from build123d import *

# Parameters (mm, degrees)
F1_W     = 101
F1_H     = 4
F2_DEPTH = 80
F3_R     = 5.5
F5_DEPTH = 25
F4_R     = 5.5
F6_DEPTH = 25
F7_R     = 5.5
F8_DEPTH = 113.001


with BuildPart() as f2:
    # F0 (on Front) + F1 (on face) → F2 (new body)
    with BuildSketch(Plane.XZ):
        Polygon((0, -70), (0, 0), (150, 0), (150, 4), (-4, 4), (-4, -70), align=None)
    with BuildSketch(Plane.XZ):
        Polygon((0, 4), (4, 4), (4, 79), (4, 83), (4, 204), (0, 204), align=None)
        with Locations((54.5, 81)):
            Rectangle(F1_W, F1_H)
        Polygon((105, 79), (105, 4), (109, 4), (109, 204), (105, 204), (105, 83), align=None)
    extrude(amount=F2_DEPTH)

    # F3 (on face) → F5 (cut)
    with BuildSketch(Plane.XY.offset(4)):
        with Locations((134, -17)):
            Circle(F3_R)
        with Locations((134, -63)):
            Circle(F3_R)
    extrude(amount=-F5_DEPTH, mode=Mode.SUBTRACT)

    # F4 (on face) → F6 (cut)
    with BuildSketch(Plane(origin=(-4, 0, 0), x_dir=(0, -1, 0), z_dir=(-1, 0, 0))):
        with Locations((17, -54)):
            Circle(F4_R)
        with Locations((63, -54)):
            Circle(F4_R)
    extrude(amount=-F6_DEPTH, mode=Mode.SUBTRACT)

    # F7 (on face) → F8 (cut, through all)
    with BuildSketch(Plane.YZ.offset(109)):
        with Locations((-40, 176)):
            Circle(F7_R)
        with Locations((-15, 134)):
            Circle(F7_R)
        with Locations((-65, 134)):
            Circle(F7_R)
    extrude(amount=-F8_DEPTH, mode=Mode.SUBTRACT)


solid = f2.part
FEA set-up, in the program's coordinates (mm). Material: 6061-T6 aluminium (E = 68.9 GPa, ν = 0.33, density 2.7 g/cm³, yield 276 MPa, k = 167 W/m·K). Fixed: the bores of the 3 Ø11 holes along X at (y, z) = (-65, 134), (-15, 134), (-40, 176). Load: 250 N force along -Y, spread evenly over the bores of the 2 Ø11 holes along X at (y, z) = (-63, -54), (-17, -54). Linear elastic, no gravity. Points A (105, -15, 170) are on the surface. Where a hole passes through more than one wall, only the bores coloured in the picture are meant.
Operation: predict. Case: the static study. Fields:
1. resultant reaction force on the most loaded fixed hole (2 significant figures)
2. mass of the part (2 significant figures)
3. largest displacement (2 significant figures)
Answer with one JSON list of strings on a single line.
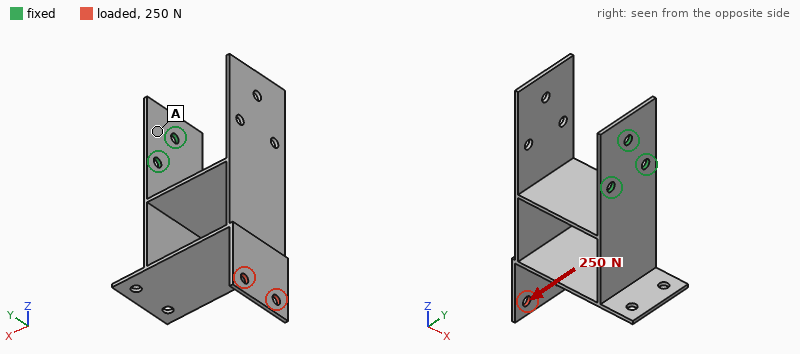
["940 N", "620 g", "3.7 mm"]
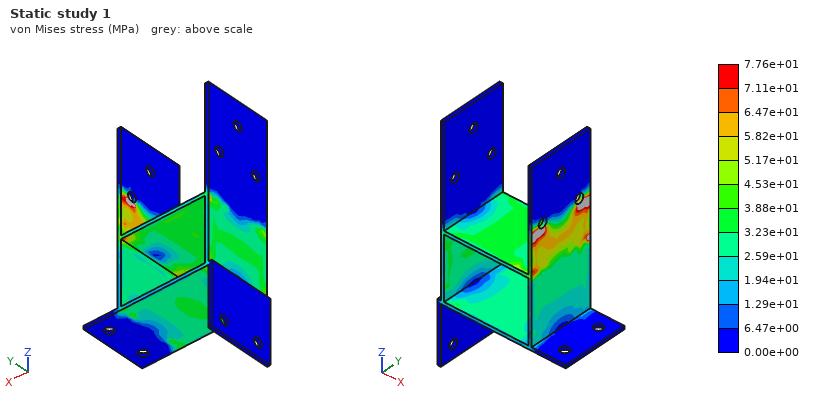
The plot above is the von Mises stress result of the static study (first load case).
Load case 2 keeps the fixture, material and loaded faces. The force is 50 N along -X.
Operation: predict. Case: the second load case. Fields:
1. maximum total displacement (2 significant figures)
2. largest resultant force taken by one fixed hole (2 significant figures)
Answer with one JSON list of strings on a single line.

["3.3 mm", "36 N"]
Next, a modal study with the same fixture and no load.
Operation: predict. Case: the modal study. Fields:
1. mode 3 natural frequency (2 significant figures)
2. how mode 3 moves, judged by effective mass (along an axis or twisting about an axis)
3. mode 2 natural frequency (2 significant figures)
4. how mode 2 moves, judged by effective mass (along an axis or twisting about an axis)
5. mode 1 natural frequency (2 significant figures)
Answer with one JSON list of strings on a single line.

["180 Hz", "along X", "120 Hz", "along Y", "44 Hz"]
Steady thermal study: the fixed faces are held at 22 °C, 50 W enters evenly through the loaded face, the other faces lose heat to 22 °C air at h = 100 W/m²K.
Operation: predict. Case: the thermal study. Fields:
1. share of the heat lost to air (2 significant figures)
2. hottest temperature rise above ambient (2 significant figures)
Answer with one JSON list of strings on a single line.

["99 %", "44 K"]
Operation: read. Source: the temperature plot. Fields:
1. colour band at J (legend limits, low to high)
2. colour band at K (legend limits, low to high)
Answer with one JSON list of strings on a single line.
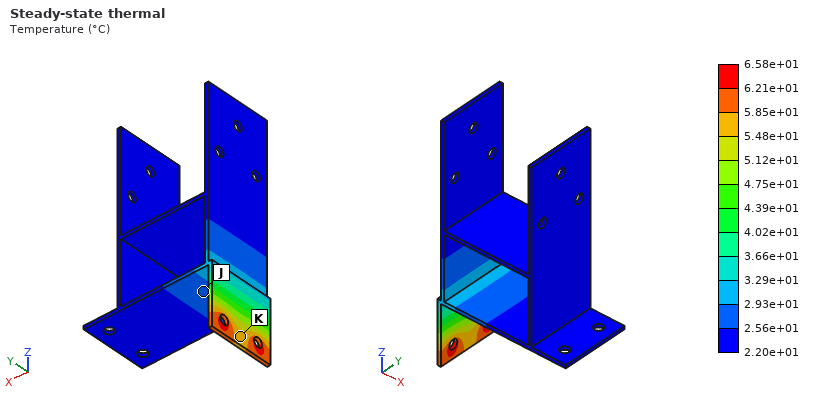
["2.56e+01 to 2.93e+01 °C", "5.48e+01 to 5.85e+01 °C"]
